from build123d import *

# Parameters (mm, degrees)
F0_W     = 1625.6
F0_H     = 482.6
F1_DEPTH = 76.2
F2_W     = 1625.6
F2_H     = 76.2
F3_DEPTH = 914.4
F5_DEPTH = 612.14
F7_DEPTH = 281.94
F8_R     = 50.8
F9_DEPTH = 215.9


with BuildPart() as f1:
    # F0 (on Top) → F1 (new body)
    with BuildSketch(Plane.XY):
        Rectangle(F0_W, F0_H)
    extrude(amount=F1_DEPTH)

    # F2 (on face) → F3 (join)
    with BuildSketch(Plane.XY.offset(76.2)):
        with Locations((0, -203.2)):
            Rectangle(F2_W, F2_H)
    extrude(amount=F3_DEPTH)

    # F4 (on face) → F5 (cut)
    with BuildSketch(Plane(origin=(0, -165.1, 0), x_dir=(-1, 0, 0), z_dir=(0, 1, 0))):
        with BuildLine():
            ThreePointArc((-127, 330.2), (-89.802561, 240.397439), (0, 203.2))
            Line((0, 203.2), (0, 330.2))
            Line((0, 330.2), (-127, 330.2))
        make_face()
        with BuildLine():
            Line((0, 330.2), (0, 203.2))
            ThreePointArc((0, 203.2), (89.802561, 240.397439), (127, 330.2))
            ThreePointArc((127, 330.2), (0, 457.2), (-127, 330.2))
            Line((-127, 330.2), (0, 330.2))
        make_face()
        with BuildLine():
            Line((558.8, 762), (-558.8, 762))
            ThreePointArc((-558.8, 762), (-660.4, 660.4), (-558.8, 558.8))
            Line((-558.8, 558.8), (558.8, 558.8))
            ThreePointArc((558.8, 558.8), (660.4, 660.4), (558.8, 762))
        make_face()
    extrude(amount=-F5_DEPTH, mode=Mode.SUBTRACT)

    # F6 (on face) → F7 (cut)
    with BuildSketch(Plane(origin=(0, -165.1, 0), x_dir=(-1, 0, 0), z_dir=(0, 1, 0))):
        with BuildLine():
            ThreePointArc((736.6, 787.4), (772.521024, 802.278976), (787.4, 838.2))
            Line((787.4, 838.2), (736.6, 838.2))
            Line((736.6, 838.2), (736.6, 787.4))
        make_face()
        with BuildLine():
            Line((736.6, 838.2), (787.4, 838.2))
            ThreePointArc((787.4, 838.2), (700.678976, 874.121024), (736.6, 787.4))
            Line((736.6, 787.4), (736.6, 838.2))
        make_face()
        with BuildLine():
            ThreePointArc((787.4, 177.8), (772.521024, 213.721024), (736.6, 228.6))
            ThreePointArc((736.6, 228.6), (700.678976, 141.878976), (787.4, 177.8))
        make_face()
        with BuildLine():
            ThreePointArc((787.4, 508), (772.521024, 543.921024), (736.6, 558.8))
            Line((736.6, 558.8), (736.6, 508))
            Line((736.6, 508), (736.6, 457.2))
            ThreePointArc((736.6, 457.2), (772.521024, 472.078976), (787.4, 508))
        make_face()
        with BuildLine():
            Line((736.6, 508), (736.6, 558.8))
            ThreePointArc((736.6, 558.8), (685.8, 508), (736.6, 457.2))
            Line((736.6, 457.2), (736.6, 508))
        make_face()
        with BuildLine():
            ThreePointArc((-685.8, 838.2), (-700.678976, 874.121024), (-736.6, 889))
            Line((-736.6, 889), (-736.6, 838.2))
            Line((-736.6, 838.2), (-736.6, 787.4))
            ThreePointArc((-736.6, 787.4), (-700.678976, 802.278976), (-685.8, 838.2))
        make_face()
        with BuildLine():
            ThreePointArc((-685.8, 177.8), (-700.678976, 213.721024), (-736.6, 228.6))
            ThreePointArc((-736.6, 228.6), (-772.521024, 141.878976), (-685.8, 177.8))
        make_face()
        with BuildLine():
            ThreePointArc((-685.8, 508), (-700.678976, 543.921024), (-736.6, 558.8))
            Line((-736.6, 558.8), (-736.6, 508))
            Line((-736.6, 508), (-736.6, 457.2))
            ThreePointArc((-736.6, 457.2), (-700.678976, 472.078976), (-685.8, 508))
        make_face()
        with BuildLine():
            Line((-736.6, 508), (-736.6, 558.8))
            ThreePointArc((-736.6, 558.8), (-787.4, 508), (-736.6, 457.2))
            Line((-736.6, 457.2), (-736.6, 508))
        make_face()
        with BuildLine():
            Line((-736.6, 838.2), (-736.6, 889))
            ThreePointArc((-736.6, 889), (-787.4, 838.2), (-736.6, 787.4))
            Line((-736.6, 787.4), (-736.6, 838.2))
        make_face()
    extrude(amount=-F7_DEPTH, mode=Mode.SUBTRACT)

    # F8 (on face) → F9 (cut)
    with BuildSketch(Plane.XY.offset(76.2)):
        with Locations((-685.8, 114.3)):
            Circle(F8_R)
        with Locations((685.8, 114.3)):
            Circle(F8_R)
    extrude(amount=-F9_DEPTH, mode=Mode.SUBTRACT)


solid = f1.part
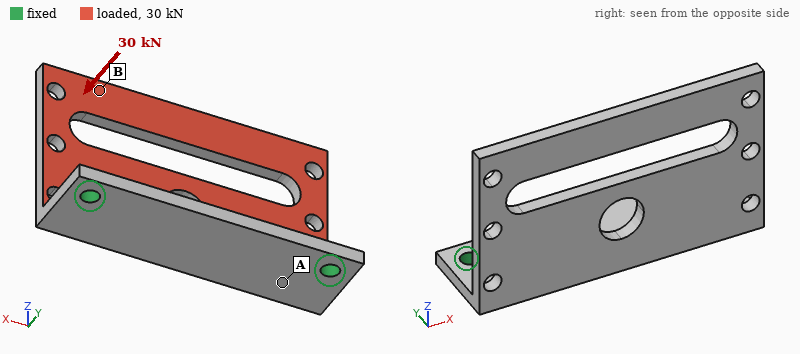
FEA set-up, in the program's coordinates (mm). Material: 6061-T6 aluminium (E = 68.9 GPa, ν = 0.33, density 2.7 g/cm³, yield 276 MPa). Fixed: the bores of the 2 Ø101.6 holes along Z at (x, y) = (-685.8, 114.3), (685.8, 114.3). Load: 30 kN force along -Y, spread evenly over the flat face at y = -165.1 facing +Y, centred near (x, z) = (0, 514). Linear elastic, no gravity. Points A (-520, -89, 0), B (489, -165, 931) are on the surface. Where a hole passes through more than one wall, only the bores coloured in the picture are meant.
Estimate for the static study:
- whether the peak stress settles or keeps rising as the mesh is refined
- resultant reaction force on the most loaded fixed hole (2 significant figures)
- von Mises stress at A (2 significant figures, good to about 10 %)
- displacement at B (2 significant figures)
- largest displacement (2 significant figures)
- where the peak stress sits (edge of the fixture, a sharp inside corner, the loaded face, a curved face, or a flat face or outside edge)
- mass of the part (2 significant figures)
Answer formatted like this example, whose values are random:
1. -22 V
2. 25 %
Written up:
1. keeps rising
2. 17 kN
3. 9.3 MPa
4. 2.7 mm
5. 3.1 mm
6. edge of the fixture
7. 390 kg
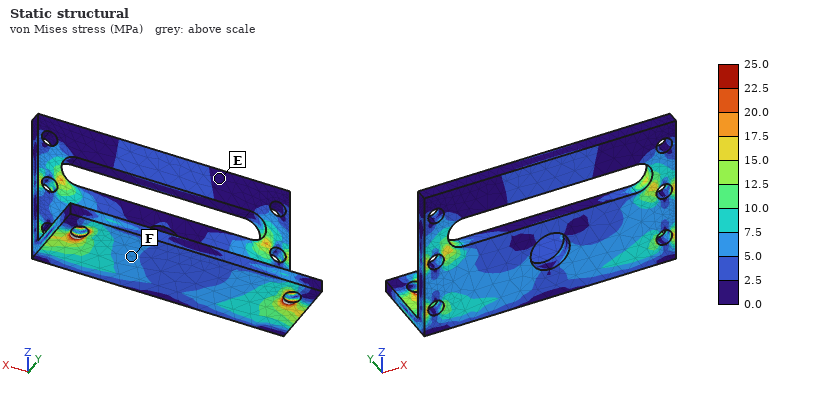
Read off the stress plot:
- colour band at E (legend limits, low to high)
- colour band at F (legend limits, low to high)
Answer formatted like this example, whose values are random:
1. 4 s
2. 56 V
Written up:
1. 0.0 to 2.5 MPa
2. 5.0 to 7.5 MPa
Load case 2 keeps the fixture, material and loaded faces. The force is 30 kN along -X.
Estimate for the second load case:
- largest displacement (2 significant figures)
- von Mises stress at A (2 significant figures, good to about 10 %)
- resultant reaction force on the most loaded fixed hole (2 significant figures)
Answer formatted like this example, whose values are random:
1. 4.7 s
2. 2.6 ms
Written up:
1. 0.26 mm
2. 1.6 MPa
3. 19 kN
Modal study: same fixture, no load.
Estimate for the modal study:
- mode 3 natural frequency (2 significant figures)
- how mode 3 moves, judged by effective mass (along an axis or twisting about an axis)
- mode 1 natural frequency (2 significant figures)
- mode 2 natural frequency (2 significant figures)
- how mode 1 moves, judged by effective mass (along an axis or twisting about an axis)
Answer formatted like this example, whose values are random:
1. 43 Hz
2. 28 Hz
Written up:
1. 130 Hz
2. along Z
3. 40 Hz
4. 89 Hz
5. along Y
